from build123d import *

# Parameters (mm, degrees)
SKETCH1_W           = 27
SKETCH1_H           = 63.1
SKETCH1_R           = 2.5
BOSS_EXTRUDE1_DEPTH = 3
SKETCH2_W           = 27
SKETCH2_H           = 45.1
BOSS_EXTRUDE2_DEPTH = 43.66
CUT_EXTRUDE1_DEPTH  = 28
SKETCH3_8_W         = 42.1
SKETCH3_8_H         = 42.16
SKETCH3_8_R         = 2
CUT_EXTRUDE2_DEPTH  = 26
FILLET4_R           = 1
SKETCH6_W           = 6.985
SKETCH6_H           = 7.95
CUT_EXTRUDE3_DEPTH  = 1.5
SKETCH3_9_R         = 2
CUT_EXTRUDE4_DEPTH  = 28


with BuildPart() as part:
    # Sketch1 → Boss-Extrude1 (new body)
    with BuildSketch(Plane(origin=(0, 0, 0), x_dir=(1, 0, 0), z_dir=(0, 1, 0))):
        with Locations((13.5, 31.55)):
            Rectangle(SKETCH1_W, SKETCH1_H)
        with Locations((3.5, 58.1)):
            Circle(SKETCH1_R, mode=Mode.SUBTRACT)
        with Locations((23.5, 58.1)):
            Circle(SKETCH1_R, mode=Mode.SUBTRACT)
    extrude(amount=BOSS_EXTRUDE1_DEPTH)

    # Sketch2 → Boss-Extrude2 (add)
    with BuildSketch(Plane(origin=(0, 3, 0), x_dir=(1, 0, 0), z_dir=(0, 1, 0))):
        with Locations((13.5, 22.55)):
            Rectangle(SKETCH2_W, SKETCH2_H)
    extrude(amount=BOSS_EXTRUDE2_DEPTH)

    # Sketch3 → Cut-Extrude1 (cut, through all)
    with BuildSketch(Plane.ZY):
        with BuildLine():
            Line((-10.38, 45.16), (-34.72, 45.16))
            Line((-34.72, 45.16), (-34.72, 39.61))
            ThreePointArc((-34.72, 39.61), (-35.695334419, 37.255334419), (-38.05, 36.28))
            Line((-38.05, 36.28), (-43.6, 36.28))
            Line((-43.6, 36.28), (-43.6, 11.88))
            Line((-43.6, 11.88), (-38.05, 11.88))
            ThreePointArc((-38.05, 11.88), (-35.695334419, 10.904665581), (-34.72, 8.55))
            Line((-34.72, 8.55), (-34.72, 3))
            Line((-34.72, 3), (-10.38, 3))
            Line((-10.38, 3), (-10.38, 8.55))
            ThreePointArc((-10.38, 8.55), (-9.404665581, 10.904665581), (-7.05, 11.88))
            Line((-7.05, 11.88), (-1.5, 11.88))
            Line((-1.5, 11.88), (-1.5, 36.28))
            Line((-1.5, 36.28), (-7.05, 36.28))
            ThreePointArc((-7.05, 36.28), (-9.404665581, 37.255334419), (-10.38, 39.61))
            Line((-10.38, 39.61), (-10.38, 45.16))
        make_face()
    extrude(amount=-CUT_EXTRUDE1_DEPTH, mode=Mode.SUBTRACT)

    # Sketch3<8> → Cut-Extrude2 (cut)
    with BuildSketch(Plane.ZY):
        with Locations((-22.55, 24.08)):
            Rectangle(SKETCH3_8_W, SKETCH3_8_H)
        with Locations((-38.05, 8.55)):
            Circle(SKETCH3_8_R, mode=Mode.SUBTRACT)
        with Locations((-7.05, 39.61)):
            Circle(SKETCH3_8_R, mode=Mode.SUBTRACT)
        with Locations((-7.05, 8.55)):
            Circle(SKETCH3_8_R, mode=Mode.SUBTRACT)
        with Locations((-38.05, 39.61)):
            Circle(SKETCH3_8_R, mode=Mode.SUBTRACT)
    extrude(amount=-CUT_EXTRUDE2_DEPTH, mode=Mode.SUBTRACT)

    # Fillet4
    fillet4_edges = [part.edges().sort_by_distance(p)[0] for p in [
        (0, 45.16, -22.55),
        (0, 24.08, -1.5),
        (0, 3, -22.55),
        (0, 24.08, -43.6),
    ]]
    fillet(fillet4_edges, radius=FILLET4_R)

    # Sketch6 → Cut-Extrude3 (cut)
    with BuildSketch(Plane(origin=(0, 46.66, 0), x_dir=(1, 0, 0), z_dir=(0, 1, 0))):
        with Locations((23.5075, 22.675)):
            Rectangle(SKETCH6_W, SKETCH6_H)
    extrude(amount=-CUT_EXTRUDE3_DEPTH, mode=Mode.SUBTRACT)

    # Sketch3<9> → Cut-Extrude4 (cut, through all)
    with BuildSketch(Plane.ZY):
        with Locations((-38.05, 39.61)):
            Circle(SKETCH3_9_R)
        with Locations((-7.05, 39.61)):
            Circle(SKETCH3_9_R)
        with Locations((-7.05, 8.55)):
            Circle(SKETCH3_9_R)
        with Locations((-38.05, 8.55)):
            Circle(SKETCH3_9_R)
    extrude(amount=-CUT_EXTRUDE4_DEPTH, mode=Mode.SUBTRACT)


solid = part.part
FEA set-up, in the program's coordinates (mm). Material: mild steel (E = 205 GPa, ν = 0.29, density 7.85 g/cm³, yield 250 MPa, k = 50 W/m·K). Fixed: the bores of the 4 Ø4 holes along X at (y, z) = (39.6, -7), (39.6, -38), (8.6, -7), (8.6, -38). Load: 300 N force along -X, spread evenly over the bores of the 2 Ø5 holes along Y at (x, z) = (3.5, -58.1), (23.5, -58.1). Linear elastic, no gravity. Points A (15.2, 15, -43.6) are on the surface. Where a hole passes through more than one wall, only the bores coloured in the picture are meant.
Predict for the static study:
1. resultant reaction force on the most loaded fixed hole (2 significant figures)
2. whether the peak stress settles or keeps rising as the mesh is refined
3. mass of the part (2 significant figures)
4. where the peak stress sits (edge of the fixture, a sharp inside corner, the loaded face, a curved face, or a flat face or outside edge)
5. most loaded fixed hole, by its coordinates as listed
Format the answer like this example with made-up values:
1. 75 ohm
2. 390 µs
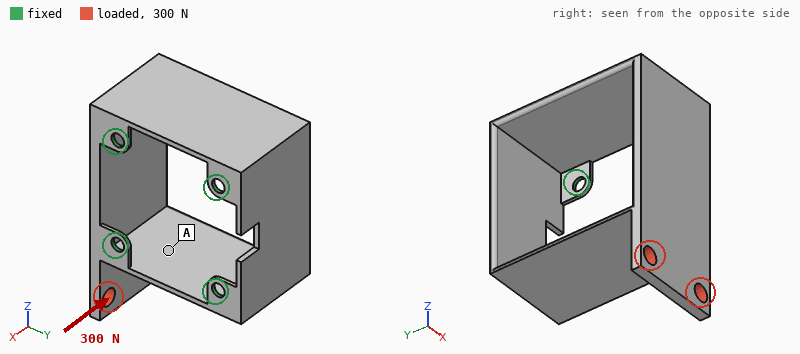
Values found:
1. 490 N
2. keeps rising
3. 81 g
4. edge of the fixture
5. (8.6, -38)
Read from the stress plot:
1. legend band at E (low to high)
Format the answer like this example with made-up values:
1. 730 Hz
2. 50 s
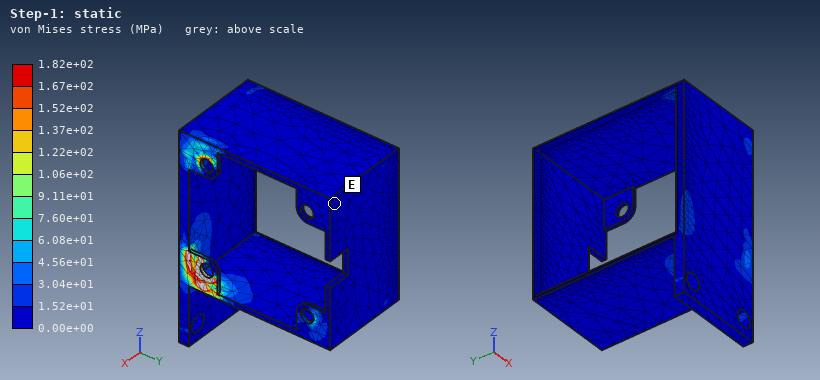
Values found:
1. 0.00e+00 to 1.52e+01 MPa
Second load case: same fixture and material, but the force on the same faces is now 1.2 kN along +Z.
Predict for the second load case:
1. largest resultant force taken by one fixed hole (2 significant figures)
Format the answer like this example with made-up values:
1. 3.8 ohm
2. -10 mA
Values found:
1. 790 N
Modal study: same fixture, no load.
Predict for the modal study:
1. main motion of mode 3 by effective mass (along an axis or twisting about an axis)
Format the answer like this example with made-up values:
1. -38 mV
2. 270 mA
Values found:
1. along Y
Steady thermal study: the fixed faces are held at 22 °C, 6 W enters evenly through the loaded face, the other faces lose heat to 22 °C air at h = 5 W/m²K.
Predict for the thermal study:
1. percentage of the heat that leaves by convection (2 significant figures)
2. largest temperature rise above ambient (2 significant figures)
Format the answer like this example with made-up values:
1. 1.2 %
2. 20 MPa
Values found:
1. 15 %
2. 61 K
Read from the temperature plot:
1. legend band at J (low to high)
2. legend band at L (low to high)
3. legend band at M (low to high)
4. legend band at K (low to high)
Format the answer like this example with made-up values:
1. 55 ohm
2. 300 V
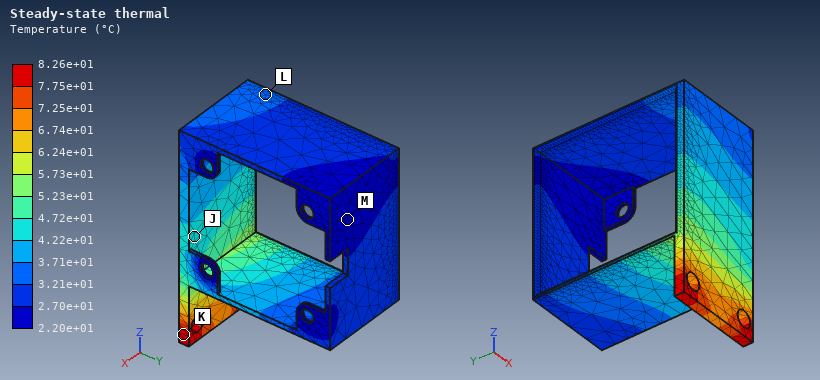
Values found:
1. 4.22e+01 to 4.72e+01 °C
2. 3.21e+01 to 3.71e+01 °C
3. 2.20e+01 to 2.70e+01 °C
4. 7.75e+01 to 8.26e+01 °C
